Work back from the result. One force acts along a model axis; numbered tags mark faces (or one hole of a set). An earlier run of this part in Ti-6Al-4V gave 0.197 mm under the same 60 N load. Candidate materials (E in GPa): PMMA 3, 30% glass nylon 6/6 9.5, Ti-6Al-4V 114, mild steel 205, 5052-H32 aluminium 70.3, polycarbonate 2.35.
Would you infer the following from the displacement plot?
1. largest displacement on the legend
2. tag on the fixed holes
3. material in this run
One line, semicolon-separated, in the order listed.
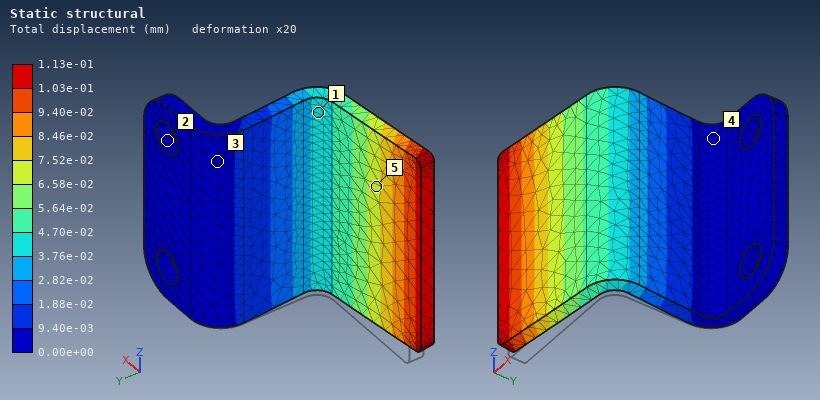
1.13e-01 mm; 2; mild steel
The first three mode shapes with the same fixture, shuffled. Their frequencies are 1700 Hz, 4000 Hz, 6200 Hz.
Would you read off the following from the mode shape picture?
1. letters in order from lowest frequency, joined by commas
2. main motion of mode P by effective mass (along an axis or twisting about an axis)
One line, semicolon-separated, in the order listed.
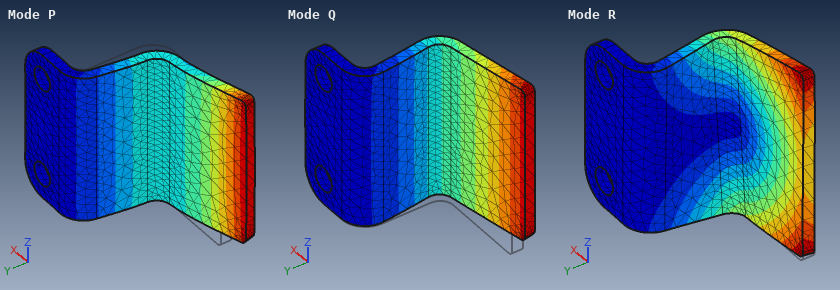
Q, R, P; along X
